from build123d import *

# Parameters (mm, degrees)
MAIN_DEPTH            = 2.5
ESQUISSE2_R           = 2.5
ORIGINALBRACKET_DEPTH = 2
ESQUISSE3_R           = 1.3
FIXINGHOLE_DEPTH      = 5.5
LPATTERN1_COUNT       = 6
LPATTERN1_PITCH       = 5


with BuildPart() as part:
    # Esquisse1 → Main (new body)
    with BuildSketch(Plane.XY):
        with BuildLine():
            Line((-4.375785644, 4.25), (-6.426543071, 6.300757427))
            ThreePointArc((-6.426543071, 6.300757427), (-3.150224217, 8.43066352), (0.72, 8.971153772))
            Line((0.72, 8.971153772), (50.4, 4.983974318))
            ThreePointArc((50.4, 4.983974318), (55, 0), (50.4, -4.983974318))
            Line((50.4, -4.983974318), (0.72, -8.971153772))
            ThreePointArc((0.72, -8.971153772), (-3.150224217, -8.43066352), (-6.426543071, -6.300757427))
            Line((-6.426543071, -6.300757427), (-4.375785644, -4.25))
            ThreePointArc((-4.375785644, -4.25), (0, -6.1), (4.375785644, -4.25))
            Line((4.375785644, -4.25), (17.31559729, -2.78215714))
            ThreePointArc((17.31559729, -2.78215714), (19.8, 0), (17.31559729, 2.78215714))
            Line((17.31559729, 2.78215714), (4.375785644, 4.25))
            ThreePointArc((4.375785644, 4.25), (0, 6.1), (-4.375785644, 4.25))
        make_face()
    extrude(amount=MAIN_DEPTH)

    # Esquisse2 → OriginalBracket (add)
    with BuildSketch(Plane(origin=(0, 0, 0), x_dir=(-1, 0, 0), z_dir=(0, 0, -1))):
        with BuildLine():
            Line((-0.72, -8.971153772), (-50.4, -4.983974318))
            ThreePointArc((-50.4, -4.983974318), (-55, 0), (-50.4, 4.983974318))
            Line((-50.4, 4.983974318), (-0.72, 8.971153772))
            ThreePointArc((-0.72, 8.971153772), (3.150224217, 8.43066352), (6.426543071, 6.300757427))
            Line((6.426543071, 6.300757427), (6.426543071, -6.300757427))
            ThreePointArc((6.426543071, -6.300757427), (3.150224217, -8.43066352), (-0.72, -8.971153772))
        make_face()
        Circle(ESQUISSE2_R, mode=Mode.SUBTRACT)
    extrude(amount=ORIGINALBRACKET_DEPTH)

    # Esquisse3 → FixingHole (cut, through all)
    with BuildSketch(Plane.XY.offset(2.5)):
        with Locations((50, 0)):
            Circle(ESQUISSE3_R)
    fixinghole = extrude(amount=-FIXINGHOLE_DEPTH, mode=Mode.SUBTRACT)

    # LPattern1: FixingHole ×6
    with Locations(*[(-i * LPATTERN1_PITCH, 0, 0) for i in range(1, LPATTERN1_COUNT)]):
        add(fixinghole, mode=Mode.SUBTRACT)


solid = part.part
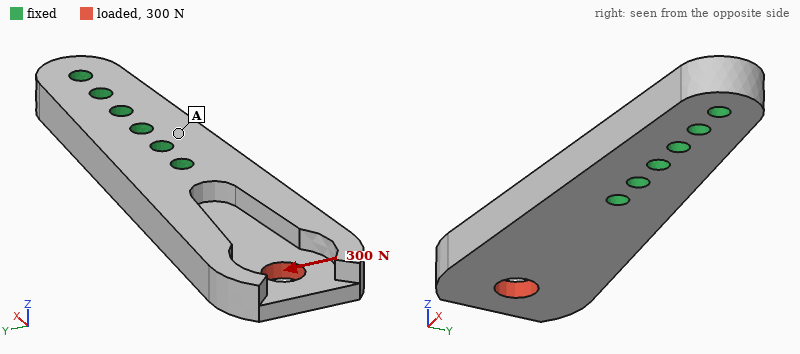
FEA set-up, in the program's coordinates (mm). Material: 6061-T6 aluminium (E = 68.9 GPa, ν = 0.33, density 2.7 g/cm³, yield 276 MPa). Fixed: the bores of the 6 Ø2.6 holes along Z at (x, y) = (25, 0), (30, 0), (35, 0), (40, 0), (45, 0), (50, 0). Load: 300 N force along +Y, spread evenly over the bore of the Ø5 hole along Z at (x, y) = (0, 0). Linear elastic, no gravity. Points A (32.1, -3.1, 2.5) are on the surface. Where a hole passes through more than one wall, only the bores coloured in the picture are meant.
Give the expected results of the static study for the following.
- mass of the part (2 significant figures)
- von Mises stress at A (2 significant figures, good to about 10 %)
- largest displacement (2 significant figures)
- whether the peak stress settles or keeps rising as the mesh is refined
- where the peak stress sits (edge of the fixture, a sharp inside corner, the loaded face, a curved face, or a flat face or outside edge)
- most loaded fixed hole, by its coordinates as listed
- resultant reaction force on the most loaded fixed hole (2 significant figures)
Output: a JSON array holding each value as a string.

["8.3 g", "17 MPa", "63 µm", "keeps rising", "edge of the fixture", "(25, 0)", "880 N"]
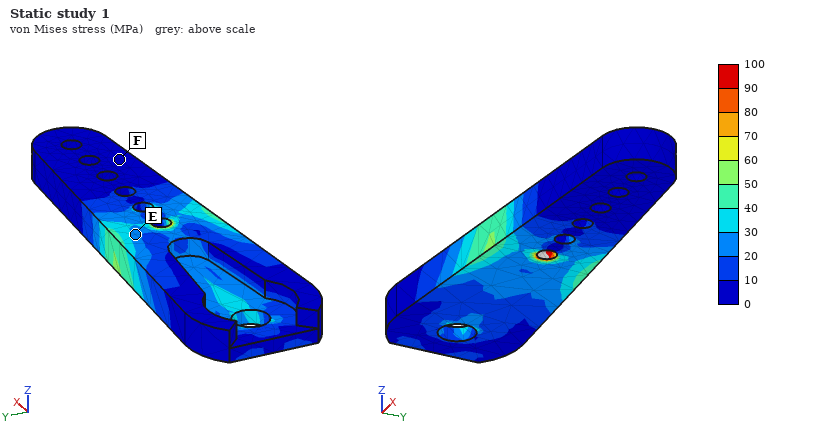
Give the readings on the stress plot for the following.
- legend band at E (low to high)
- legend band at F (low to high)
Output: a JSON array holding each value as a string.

["20 to 30 MPa", "0 to 10 MPa"]
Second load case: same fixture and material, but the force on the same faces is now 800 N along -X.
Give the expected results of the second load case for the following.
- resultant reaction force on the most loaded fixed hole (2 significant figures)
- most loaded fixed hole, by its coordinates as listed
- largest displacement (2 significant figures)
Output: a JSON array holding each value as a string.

["540 N", "(25, 0)", "59 µm"]
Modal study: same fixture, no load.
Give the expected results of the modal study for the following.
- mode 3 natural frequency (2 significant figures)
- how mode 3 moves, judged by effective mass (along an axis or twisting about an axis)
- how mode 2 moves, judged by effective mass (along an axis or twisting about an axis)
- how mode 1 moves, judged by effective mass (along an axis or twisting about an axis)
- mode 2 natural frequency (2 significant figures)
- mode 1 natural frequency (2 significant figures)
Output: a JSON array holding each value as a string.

["9600 Hz", "along Y", "along Y", "along Z", "8000 Hz", "4000 Hz"]
